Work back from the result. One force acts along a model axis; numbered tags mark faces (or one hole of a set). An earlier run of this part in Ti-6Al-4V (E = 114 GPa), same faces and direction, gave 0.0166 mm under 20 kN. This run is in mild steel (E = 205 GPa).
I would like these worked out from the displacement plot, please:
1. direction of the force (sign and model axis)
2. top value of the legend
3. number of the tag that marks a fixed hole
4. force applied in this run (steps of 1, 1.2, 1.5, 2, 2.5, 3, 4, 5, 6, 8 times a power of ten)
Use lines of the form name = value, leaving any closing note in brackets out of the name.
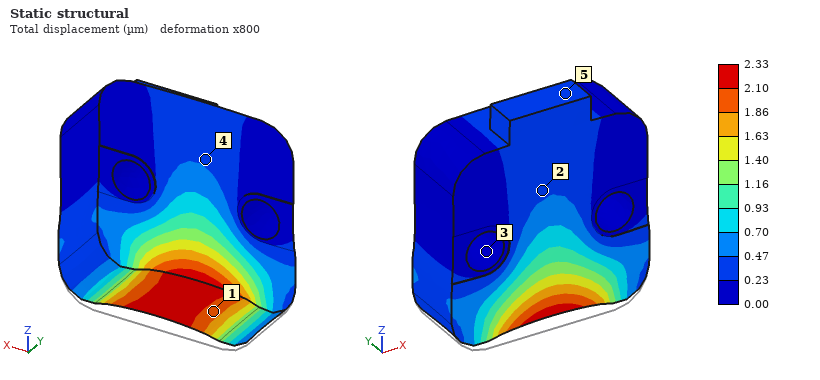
direction of the force = +Z
top value of the legend = 2.33 µm
number of the tag that marks a fixed hole = 3
force applied in this run = 5 kN
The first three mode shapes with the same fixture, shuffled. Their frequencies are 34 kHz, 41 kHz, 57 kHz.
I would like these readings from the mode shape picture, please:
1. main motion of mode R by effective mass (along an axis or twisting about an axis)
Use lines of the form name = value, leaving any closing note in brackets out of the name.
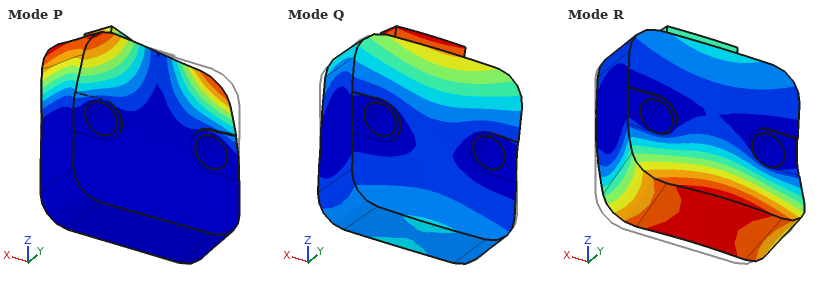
main motion of mode R by effective mass = along Y
